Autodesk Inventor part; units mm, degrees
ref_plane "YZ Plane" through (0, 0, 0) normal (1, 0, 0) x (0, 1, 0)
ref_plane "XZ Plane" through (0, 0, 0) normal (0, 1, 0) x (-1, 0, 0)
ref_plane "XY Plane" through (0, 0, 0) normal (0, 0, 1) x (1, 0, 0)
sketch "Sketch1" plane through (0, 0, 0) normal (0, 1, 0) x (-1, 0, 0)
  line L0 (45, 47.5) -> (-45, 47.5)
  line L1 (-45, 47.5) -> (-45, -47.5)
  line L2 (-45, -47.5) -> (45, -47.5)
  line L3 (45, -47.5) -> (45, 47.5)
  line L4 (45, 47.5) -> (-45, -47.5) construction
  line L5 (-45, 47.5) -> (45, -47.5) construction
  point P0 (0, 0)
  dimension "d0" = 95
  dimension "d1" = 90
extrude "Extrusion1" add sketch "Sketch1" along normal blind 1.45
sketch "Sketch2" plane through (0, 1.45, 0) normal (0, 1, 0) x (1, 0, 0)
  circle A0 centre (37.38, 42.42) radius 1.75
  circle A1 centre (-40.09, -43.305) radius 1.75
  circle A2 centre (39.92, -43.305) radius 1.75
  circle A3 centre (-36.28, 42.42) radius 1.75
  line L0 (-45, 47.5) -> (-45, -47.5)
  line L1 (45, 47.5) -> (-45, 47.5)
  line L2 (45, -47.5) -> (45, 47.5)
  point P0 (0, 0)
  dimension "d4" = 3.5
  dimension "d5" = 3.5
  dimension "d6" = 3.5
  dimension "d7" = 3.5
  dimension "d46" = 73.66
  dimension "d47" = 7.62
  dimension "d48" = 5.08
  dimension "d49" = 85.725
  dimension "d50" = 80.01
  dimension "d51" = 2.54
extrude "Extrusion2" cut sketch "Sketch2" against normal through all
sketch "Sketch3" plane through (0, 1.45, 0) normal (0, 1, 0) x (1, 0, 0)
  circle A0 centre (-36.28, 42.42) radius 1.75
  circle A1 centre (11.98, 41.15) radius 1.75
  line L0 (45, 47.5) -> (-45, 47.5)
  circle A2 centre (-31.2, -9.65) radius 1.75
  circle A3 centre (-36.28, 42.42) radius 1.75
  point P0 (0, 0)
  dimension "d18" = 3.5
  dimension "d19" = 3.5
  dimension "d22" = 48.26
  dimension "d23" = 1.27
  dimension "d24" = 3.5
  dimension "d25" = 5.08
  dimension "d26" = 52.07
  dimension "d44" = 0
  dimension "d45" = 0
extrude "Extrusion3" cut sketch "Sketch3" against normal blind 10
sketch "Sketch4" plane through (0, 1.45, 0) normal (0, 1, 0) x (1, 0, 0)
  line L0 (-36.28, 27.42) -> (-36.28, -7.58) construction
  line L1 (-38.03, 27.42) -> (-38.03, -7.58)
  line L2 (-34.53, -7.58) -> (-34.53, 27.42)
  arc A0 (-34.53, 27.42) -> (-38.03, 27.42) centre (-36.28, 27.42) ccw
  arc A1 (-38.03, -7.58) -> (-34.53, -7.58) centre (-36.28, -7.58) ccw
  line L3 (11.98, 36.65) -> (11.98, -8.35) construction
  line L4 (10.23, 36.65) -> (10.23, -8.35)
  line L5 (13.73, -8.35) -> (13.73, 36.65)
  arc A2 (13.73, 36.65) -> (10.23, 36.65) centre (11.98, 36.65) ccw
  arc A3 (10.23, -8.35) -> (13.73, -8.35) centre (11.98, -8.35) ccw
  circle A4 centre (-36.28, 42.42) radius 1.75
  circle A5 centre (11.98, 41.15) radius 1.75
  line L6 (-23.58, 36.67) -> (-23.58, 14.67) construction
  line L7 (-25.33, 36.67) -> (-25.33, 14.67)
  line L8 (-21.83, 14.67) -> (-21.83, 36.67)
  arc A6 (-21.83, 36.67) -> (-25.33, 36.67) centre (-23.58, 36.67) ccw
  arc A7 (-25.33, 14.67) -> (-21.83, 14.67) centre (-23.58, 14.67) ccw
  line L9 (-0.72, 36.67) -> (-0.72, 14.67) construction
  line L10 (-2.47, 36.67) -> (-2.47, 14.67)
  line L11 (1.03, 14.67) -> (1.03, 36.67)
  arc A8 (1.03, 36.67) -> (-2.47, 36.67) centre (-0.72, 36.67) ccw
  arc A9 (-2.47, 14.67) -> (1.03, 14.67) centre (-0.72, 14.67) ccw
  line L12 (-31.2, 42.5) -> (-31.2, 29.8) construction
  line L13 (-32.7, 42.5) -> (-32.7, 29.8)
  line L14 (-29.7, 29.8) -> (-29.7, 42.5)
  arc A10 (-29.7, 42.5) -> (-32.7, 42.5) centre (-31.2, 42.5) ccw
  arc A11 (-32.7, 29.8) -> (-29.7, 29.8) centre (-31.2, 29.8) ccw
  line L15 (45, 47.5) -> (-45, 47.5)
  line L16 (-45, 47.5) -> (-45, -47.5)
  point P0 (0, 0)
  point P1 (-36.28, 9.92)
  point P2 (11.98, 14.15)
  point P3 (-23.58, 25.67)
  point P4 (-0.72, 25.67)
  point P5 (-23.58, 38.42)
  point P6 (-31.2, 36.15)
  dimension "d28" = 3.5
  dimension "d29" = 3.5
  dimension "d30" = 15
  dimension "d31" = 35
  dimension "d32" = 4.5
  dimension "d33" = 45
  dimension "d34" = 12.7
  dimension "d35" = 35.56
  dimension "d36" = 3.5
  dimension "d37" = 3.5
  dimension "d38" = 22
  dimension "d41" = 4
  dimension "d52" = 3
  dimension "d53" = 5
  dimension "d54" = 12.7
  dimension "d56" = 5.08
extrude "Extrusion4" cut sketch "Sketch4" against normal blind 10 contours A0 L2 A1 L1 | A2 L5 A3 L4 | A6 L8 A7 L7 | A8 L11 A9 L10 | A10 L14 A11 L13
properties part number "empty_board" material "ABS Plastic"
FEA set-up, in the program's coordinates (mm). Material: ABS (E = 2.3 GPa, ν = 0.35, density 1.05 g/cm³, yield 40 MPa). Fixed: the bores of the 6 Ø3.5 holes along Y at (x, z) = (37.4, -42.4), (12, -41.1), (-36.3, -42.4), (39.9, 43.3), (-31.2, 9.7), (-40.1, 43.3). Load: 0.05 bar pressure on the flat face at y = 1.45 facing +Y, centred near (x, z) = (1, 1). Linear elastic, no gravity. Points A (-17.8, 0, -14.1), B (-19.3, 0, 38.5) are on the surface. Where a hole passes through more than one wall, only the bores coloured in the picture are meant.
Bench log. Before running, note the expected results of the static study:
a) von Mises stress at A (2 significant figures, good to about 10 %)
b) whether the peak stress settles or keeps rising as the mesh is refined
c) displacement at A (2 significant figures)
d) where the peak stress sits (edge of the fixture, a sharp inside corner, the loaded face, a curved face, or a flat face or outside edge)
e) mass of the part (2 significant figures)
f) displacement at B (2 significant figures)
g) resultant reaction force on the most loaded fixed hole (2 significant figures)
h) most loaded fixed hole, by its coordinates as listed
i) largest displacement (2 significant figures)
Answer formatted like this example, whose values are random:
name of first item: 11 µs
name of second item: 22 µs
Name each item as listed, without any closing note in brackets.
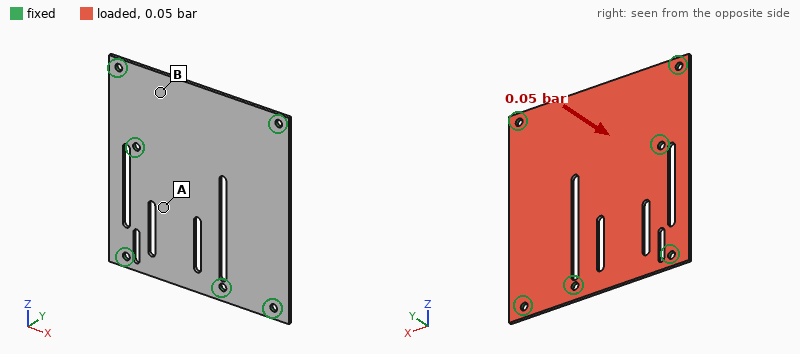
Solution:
von Mises stress at A: 2.9 MPa
whether the peak stress settles or keeps rising as the mesh is refined: keeps rising
displacement at A: 0.52 mm
where the peak stress sits: edge of the fixture
mass of the part: 12 g
displacement at B: 0.48 mm
resultant reaction force on the most loaded fixed hole: 12 N
most loaded fixed hole, by its coordinates as listed: (-31.2, 9.7)
largest displacement: 1.4 mm
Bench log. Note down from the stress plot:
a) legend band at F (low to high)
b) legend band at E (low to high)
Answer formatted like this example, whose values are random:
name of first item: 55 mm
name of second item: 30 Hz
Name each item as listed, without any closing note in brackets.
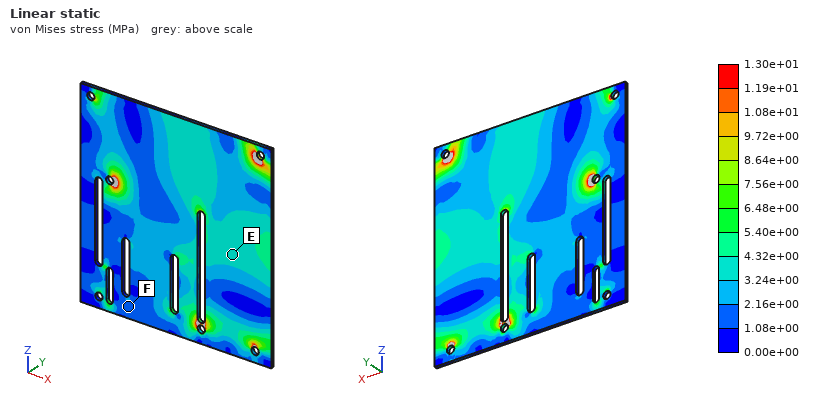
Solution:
legend band at F: 1.08e+00 to 2.16e+00 MPa
legend band at E: 3.24e+00 to 4.32e+00 MPa
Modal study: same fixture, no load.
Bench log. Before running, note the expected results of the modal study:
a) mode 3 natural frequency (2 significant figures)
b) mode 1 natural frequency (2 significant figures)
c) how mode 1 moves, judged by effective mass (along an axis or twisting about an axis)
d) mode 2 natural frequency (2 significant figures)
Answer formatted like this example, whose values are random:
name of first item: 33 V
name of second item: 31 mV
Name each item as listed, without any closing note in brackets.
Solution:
mode 3 natural frequency: 500 Hz
mode 1 natural frequency: 290 Hz
how mode 1 moves, judged by effective mass: along Y
mode 2 natural frequency: 400 Hz
